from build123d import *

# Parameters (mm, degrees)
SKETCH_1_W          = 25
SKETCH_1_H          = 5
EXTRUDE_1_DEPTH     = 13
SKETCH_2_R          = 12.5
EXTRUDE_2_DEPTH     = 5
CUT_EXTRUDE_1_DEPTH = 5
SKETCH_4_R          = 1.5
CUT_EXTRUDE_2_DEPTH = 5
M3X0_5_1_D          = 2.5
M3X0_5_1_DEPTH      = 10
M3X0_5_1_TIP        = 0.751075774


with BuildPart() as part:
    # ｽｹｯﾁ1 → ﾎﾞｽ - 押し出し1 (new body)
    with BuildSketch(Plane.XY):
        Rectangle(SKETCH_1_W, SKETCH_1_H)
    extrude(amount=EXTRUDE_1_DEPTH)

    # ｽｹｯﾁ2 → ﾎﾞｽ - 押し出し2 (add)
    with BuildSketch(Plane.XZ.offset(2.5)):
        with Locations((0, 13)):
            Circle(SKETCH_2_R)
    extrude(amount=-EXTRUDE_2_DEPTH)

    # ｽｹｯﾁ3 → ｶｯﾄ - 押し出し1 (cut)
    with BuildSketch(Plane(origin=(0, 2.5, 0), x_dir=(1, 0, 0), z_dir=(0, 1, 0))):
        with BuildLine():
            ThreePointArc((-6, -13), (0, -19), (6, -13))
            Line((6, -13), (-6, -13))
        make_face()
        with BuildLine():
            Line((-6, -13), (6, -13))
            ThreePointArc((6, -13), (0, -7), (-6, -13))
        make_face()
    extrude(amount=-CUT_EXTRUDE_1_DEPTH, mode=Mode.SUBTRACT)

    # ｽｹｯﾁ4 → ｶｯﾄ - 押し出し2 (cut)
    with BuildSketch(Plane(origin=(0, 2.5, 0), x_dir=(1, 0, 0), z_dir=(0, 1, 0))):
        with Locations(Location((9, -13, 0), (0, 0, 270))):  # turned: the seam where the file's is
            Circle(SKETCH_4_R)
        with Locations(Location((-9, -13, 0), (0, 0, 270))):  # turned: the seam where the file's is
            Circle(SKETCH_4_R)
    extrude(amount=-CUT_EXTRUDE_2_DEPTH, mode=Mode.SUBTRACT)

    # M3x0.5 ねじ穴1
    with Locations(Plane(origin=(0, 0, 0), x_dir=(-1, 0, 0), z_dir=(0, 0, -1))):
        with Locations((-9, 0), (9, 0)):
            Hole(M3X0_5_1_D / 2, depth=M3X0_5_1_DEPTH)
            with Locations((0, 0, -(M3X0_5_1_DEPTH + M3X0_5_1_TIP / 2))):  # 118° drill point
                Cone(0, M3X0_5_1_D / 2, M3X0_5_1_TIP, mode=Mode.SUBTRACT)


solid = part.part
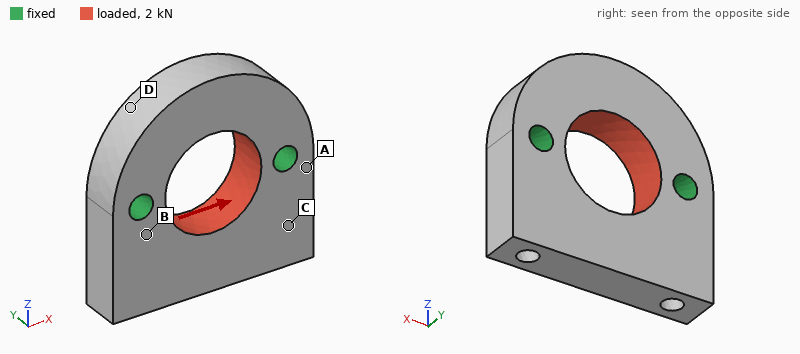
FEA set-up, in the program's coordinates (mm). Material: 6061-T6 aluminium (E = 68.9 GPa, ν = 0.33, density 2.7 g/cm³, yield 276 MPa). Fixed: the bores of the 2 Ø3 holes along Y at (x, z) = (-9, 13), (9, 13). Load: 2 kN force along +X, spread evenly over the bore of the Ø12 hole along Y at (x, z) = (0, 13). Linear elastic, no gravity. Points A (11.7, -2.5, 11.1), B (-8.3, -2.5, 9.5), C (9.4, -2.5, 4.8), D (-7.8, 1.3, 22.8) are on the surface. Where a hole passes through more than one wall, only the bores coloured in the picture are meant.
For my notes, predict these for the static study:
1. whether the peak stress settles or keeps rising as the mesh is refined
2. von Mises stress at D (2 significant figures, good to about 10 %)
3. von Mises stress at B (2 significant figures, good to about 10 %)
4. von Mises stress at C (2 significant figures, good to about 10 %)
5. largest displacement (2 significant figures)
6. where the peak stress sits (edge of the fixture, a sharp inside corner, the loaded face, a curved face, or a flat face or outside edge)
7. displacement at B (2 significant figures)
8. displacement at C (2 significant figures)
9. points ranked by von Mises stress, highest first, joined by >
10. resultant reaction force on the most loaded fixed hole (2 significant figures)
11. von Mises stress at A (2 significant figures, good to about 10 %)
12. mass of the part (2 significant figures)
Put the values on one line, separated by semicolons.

keeps rising; 11 MPa; 23 MPa; 4.5 MPa; 4.7 µm; edge of the fixture; 1.8 µm; 3.4 µm; B > A > D > C; 1.0 kN; 17 MPa; 5.7 g
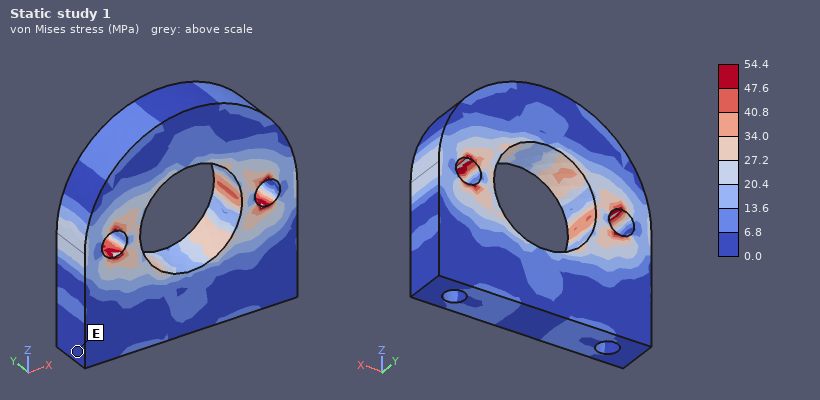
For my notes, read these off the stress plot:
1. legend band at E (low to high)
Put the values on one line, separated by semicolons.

0.0 to 6.8 MPa
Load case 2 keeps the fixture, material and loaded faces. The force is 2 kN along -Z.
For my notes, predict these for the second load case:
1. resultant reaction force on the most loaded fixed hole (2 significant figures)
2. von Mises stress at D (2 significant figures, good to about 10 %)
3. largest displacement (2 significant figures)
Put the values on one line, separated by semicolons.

1.0 kN; 7.8 MPa; 3.7 µm
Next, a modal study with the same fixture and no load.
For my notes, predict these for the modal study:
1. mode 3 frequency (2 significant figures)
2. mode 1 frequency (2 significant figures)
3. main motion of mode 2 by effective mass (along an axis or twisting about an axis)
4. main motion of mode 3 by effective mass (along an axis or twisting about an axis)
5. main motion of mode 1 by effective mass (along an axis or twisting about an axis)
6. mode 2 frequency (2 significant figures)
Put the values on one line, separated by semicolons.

31 kHz; 18 kHz; along Y; twisting about Z; along Y; 23 kHz
